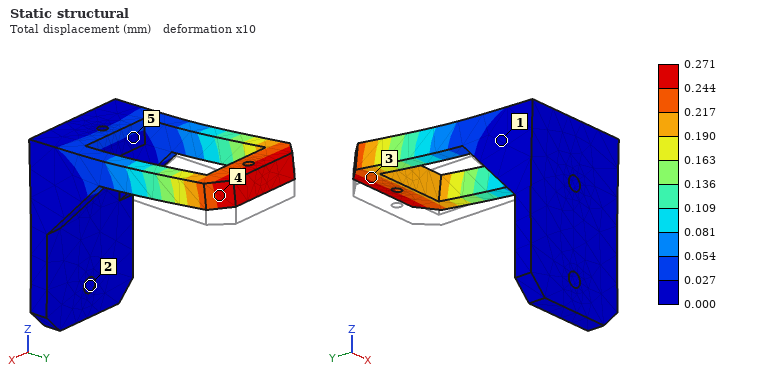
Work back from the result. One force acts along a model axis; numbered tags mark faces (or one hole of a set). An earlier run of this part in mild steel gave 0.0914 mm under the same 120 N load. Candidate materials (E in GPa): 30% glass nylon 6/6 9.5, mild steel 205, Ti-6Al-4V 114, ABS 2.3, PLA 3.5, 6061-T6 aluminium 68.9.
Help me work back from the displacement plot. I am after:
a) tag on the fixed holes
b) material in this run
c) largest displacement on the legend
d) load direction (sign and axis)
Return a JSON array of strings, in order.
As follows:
["2", "6061-T6 aluminium", "0.271 mm", "+Z"]
